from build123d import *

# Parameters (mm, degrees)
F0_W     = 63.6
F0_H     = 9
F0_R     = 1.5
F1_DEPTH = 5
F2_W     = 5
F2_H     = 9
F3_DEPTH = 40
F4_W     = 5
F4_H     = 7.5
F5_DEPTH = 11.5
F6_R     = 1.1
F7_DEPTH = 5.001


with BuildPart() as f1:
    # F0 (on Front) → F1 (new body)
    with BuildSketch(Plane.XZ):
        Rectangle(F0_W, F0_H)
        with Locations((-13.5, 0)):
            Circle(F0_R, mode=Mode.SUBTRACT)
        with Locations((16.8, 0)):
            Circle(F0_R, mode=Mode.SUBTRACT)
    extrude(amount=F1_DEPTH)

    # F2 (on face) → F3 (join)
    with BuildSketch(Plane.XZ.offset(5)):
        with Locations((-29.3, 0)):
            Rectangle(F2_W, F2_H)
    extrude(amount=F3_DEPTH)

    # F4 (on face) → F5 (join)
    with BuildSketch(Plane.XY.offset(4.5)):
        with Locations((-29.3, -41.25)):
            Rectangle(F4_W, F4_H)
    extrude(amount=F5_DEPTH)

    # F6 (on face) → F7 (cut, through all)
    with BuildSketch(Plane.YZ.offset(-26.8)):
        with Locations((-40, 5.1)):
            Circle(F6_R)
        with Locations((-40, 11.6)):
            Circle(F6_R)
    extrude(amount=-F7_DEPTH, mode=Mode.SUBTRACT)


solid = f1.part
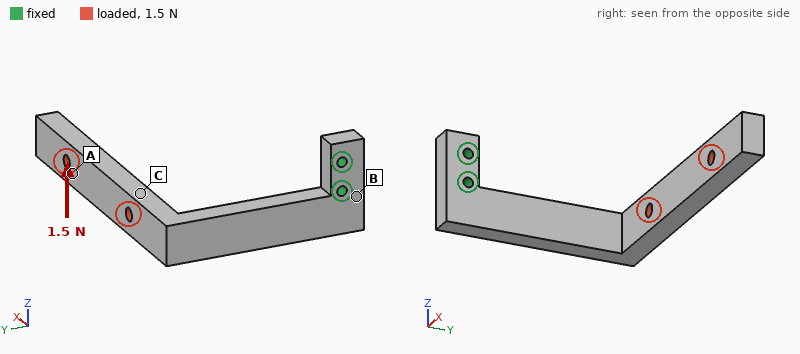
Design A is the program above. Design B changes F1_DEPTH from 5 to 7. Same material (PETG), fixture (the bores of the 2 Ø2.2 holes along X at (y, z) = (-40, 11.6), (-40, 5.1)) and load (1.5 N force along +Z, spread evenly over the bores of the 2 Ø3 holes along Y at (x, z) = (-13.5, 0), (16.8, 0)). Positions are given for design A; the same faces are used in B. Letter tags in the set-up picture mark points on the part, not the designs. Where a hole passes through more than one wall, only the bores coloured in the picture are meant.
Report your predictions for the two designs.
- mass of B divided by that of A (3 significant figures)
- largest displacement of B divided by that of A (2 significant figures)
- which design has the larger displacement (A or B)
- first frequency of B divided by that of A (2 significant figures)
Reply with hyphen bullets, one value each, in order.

- 1.21
- 0.91
- A
- 0.92
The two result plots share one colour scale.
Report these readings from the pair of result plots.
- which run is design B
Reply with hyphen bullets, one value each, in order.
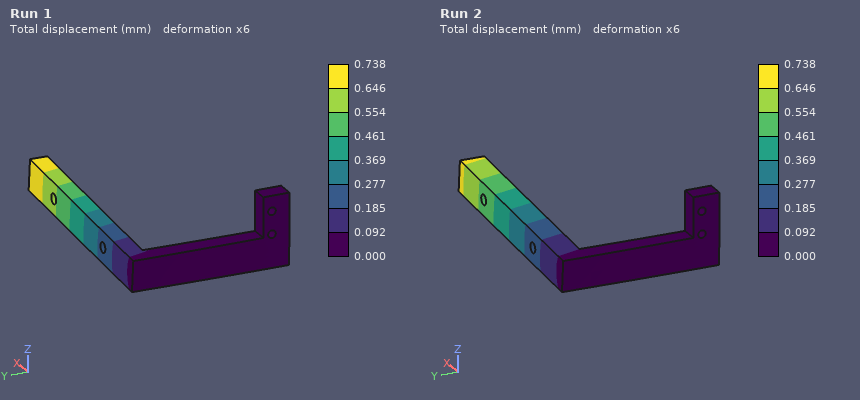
- Run 2
